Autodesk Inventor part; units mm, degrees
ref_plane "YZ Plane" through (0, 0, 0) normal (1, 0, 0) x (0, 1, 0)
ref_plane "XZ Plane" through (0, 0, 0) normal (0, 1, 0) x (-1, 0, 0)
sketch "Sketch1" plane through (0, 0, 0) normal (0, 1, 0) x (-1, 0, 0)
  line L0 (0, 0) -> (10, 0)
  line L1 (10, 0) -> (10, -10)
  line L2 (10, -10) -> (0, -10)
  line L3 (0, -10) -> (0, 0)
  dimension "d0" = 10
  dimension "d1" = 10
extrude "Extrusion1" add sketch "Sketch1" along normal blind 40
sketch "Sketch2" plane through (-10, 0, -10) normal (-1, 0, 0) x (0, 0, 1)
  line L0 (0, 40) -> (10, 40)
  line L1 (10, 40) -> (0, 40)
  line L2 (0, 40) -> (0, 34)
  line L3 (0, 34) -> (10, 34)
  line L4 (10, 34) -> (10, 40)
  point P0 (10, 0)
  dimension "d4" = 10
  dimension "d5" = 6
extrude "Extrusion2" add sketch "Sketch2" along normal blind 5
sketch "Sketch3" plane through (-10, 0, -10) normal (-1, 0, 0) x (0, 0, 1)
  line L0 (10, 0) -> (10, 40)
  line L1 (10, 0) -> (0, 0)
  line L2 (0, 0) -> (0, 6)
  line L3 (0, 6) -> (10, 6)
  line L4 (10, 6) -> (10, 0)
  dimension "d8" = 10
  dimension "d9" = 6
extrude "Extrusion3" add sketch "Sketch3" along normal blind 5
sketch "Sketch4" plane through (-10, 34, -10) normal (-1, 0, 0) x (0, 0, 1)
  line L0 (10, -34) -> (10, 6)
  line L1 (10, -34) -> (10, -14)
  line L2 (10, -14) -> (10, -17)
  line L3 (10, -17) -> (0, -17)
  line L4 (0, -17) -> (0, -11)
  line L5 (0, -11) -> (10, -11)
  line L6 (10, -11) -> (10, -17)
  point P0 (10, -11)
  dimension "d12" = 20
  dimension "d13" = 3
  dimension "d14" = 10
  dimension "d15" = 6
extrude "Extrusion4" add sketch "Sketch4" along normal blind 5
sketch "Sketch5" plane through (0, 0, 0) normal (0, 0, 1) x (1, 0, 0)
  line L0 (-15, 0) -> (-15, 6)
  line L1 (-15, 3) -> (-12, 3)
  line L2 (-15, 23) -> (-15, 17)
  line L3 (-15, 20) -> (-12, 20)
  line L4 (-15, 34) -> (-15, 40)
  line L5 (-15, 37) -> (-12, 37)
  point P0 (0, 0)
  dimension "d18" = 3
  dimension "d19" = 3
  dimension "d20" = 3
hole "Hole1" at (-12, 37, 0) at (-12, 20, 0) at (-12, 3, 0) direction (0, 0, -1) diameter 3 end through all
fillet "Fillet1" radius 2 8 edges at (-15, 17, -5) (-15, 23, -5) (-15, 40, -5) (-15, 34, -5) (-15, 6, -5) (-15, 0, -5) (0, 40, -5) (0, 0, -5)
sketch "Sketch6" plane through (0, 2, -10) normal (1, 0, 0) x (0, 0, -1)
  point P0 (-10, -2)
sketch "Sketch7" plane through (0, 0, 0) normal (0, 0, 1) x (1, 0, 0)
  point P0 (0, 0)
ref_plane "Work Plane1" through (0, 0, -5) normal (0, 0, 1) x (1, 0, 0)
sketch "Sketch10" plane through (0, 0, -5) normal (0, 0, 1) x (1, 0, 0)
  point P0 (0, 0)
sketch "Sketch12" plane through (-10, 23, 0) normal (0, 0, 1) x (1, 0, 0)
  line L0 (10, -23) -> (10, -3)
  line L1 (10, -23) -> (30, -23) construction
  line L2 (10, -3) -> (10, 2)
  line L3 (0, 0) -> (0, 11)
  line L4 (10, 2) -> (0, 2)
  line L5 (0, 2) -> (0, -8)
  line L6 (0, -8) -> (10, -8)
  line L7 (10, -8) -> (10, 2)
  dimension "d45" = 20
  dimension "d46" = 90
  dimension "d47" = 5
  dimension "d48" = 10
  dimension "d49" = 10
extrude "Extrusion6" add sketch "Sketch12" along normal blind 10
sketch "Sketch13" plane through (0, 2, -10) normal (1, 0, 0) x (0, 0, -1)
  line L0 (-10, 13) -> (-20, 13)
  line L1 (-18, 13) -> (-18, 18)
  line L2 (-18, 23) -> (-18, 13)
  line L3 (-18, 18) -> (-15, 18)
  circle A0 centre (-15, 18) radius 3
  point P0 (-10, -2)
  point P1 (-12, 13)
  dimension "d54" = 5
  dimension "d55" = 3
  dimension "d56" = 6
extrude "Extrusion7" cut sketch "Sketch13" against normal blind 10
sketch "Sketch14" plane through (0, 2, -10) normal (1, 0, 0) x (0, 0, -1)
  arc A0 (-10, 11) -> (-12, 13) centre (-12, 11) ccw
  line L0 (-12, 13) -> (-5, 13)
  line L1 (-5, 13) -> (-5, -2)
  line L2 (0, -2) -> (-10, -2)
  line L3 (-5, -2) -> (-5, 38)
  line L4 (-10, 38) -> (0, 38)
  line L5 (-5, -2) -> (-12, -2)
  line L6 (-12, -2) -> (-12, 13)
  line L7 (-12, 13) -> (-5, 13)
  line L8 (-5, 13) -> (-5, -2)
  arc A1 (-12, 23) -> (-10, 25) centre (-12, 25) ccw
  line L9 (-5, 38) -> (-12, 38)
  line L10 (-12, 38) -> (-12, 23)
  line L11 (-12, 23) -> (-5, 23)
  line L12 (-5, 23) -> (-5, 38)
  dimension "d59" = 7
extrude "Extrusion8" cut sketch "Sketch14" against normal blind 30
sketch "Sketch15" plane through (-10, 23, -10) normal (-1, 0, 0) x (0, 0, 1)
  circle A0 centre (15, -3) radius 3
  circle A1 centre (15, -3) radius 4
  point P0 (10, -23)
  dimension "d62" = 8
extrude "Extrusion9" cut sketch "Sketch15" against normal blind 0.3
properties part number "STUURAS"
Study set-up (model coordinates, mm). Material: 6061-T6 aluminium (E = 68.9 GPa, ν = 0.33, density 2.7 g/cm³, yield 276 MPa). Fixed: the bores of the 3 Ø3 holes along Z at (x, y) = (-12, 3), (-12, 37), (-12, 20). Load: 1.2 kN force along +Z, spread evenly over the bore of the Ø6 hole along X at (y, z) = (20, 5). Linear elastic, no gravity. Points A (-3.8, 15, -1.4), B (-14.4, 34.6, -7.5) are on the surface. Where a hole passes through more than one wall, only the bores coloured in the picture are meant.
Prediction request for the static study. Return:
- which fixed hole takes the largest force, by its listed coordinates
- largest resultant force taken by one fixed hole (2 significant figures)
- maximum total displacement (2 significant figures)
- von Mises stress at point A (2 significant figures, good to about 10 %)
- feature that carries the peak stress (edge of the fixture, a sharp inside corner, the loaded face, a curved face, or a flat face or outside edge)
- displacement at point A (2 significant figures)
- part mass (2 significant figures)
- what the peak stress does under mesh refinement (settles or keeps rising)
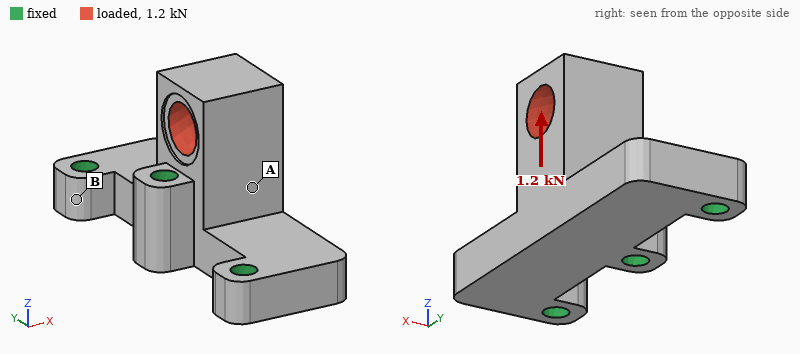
(-12, 20)
1.1 kN
17 µm
19 MPa
edge of the fixture
7.2 µm
9.8 g
keeps rising
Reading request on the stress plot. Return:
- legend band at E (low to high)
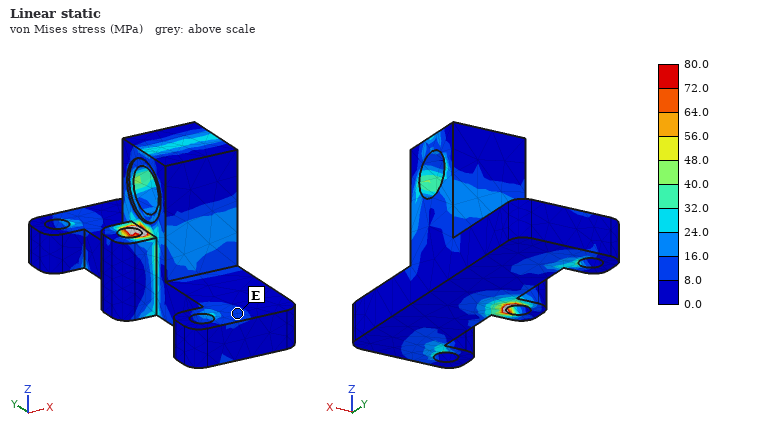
8.0 to 16.0 MPa
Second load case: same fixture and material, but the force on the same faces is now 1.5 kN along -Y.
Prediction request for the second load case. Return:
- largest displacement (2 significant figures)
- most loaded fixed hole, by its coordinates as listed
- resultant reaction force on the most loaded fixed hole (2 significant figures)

67 µm
(-12, 20)
1.1 kN
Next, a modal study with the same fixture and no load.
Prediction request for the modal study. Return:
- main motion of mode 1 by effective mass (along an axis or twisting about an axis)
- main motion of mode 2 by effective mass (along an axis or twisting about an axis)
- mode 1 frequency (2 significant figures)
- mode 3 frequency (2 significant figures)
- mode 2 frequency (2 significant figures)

along Y
along Z
19 kHz
33 kHz
20 kHz
